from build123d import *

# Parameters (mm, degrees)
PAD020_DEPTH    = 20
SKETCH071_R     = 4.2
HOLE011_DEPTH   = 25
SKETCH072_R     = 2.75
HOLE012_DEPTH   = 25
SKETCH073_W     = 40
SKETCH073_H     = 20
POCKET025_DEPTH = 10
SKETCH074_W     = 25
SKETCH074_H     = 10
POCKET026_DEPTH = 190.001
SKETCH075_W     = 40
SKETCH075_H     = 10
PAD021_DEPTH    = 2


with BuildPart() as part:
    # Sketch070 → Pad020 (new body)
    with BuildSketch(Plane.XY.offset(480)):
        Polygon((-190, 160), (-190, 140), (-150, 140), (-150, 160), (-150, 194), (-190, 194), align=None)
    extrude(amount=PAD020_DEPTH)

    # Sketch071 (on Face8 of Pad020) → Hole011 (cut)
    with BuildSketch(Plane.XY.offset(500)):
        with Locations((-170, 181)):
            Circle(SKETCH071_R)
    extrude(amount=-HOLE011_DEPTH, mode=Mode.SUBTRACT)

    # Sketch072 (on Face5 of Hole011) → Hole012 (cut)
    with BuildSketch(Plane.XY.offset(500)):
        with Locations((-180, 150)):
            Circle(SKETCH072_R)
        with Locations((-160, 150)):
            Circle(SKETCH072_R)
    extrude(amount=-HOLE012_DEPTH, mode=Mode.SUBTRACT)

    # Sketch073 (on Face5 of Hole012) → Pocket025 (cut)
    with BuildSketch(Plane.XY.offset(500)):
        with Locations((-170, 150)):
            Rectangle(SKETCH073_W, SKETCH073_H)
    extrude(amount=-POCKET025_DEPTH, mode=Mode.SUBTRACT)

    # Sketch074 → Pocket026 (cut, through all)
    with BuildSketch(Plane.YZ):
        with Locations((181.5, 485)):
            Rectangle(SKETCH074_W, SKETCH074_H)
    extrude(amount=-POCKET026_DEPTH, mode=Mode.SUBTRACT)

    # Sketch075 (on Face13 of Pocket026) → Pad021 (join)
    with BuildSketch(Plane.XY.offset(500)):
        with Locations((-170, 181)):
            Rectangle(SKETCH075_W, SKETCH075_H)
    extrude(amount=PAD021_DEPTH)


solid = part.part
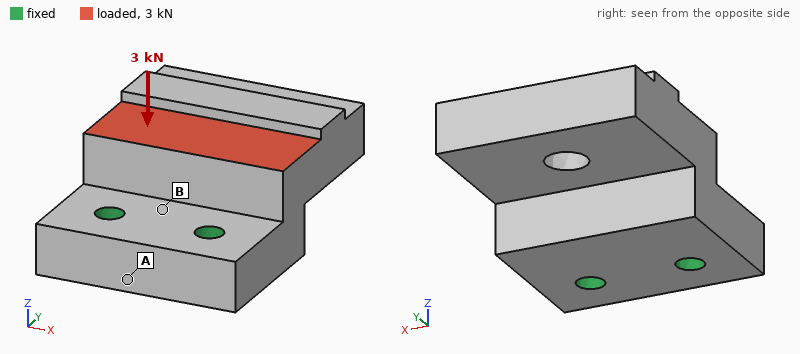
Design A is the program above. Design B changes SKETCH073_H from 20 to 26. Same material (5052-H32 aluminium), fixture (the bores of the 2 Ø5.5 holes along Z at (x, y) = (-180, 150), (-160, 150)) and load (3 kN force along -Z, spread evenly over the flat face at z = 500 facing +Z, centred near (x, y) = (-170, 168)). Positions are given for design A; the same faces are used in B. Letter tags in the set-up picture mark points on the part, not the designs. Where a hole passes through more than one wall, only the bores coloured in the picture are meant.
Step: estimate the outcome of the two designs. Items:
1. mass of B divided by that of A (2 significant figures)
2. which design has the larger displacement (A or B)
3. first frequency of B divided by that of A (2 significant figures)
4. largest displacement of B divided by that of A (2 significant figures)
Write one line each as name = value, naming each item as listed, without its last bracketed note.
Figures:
mass of B divided by that of A = 0.95
which design has the larger displacement = B
first frequency of B divided by that of A = 0.89
largest displacement of B divided by that of A = 1.3
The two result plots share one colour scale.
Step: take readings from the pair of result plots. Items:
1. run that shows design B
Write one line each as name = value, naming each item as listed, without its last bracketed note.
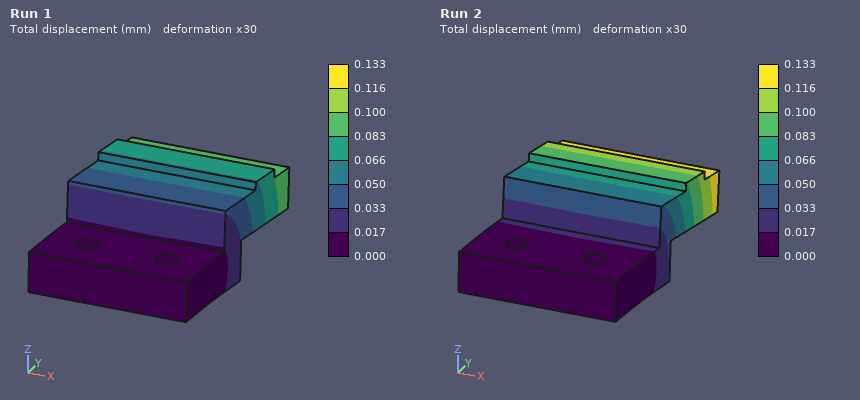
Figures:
run that shows design B = Run 2
